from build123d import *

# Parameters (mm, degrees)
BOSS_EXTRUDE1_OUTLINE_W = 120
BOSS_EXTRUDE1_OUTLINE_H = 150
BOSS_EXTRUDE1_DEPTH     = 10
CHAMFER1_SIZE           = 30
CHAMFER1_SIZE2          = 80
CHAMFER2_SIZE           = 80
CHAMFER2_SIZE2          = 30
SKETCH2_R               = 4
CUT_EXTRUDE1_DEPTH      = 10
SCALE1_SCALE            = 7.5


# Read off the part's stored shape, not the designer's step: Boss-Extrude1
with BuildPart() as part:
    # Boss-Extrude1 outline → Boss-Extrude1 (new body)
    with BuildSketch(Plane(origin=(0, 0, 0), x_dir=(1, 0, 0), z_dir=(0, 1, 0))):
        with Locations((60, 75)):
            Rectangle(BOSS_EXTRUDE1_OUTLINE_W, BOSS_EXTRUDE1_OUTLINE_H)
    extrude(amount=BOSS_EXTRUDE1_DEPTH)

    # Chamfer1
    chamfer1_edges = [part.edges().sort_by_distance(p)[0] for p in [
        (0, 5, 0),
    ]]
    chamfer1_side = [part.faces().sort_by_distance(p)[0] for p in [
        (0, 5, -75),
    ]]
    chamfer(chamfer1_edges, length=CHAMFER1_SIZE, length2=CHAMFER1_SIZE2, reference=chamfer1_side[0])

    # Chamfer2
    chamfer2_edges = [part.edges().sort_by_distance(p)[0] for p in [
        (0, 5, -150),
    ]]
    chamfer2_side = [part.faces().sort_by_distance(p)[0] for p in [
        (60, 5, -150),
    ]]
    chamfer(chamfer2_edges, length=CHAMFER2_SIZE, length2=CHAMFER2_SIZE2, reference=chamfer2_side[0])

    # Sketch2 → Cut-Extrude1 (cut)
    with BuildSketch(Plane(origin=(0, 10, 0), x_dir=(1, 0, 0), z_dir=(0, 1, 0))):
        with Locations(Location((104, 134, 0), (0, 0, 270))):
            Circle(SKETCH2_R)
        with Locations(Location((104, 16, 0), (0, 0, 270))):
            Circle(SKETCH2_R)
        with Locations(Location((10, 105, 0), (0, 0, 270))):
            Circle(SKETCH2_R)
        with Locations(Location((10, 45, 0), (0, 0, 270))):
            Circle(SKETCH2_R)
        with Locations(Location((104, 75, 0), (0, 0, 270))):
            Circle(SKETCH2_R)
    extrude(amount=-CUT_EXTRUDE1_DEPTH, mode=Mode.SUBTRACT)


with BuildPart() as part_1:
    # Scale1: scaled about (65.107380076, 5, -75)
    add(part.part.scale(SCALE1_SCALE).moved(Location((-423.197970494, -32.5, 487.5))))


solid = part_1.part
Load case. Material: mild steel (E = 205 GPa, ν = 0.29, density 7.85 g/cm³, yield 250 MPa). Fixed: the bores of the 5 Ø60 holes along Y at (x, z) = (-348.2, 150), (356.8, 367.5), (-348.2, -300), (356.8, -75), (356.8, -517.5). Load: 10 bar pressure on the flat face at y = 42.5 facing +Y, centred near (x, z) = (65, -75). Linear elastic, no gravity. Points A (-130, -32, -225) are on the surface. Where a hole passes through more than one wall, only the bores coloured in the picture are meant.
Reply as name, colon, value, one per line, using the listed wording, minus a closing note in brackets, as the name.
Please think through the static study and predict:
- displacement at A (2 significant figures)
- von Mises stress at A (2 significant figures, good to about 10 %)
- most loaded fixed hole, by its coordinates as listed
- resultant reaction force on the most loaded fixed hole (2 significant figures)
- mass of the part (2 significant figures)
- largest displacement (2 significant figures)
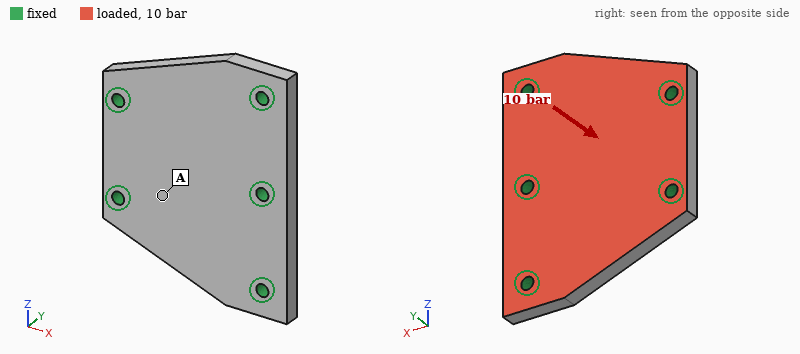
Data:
displacement at A: 0.100 mm
von Mises stress at A: 16 MPa
most loaded fixed hole, by its coordinates as listed: (356.8, -75)
resultant reaction force on the most loaded fixed hole: 210 kN
mass of the part: 510 kg
largest displacement: 0.14 mm
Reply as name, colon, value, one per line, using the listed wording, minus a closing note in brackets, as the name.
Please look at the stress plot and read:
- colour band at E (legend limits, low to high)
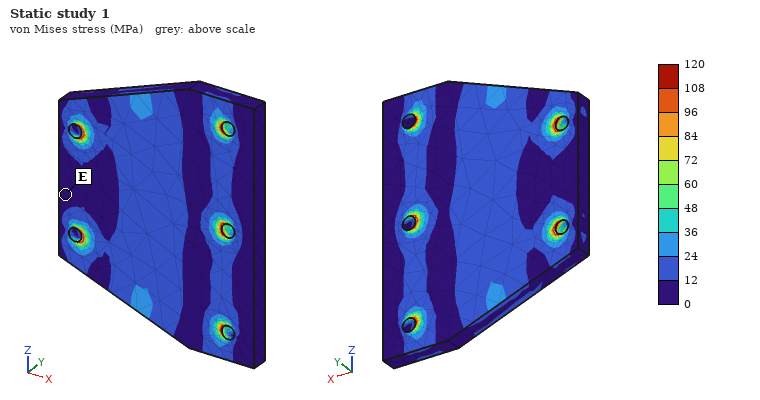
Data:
colour band at E: 0 to 12 MPa
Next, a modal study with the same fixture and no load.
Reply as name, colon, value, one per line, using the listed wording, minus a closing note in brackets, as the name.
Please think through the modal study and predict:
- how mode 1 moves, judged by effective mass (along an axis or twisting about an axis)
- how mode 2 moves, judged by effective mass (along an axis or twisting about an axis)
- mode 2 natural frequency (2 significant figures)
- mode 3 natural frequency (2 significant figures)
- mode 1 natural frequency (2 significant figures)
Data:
how mode 1 moves, judged by effective mass: along Y
how mode 2 moves, judged by effective mass: twisting about X
mode 2 natural frequency: 710 Hz
mode 3 natural frequency: 940 Hz
mode 1 natural frequency: 640 Hz
